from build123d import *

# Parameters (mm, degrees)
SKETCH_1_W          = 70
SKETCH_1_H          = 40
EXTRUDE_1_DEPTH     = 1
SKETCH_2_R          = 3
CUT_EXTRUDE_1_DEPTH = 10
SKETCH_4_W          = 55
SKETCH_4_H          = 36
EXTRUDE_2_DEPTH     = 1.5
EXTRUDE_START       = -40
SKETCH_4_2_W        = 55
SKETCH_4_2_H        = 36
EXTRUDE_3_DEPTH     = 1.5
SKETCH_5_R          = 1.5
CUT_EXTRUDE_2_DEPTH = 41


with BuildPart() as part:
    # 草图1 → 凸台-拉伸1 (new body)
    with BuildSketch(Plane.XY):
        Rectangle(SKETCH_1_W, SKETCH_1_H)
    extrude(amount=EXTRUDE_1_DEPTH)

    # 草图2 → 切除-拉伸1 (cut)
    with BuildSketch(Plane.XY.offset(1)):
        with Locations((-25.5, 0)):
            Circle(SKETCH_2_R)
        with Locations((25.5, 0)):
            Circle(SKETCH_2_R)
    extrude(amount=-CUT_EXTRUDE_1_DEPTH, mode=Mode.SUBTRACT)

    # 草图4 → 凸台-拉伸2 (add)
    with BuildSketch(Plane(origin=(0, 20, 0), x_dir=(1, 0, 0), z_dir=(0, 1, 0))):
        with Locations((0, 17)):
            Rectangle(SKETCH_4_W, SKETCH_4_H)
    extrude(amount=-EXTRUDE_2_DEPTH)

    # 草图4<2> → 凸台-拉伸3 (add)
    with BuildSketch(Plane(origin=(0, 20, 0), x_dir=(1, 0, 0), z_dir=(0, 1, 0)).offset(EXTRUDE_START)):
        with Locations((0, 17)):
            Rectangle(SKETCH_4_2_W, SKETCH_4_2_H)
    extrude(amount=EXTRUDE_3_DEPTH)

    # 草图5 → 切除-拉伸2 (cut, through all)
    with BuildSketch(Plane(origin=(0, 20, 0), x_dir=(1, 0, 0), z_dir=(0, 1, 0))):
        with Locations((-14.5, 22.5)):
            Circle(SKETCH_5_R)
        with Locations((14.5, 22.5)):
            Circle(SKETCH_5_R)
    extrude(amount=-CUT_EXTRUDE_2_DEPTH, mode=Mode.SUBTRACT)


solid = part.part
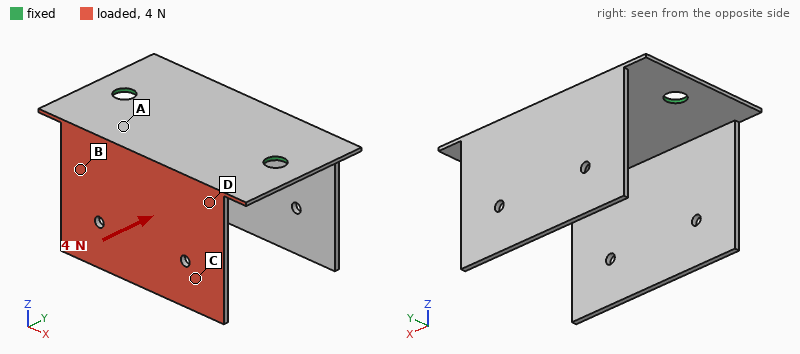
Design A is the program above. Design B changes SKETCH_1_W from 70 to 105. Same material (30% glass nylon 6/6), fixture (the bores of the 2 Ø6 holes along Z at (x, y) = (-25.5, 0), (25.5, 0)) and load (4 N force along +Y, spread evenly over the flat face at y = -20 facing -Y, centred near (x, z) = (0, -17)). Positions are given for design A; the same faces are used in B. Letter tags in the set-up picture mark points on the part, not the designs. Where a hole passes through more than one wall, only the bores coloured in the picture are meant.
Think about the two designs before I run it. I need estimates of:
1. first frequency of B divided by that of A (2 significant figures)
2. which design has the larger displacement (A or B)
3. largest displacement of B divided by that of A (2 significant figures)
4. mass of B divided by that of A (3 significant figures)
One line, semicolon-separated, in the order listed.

1.0; A; 0.89; 1.17
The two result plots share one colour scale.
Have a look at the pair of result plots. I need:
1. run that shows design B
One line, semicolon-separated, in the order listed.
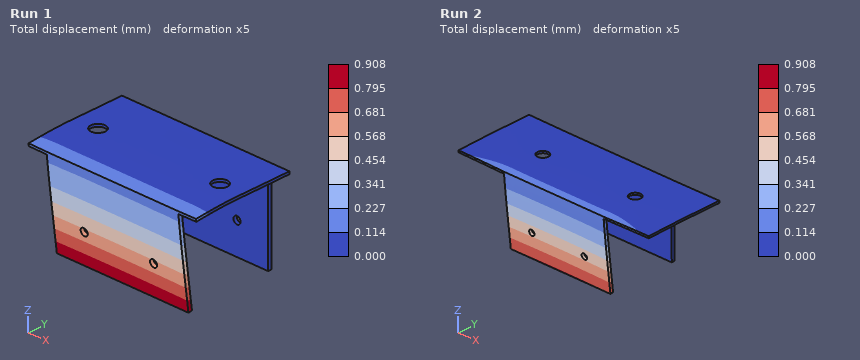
Run 2
